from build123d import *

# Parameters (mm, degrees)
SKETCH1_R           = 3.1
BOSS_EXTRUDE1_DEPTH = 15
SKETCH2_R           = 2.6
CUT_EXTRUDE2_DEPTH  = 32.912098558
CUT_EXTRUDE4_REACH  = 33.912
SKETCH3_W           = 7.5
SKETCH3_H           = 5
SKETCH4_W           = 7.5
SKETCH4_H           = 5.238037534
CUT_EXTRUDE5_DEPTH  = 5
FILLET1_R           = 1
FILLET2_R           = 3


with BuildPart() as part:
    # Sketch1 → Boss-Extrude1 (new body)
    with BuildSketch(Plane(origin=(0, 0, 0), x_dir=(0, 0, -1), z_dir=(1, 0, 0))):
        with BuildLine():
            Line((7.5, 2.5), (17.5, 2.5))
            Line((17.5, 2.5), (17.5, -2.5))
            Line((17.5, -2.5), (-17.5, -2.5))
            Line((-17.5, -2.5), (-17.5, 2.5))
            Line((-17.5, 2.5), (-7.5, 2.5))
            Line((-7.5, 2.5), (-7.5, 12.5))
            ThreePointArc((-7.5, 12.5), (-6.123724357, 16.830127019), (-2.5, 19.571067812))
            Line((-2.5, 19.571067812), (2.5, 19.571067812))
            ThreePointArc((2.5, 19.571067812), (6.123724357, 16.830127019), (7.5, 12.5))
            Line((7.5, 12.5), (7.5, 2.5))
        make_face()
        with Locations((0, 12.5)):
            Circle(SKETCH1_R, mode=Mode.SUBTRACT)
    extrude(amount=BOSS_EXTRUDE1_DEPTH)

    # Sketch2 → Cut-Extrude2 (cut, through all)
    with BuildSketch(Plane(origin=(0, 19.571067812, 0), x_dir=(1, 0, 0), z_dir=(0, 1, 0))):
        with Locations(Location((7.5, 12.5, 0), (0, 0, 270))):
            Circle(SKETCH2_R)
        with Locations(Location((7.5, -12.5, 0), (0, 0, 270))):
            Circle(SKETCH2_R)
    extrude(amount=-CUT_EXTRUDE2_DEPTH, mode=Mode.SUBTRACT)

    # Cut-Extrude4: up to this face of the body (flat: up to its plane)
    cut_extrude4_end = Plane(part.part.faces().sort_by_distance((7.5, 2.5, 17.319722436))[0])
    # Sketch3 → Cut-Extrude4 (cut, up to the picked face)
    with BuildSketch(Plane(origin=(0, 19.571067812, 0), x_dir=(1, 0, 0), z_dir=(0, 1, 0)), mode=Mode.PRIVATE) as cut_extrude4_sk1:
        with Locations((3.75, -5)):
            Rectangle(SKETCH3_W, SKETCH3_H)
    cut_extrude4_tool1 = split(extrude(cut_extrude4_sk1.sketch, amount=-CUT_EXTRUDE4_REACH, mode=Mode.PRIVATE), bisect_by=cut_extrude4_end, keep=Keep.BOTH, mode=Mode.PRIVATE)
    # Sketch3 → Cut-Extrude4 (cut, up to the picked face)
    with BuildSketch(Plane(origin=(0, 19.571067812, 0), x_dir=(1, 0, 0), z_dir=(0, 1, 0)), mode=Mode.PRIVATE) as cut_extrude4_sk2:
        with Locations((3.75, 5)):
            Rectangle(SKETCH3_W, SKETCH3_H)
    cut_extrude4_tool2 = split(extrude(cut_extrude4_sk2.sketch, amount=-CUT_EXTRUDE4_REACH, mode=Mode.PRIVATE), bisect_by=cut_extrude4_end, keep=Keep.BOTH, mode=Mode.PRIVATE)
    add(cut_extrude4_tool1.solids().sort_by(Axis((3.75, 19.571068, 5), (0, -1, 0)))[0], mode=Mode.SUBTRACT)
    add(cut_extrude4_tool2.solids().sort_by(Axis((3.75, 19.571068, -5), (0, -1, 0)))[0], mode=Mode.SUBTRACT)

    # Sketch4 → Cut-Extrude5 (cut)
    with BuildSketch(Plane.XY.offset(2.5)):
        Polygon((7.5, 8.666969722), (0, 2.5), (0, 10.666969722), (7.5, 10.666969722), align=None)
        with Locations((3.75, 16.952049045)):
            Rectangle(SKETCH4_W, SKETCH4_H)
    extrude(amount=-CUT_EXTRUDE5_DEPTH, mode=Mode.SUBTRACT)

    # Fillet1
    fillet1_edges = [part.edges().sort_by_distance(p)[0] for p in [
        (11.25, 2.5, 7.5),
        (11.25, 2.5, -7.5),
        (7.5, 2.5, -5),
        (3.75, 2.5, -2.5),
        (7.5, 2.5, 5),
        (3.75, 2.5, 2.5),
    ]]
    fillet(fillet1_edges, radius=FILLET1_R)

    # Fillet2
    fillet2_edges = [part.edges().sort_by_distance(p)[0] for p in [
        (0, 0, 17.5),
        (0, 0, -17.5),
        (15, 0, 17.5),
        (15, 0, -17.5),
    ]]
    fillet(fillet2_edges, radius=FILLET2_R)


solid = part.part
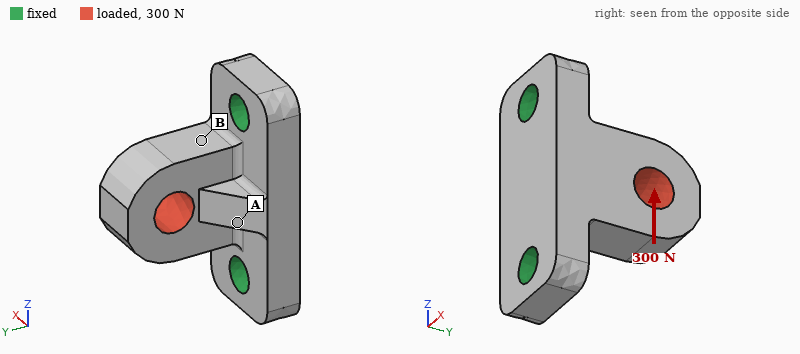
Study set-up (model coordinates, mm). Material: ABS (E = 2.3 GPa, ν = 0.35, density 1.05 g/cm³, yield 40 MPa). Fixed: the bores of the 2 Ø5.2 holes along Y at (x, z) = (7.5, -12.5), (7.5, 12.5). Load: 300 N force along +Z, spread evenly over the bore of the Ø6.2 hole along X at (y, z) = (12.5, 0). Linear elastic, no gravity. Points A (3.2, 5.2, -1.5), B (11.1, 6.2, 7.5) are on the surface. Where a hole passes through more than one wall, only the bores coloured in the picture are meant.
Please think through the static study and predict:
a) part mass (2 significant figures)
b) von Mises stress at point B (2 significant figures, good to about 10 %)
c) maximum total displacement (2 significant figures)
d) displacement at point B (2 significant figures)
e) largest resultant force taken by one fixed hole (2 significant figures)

4.3 g
9.1 MPa
0.19 mm
0.068 mm
250 N
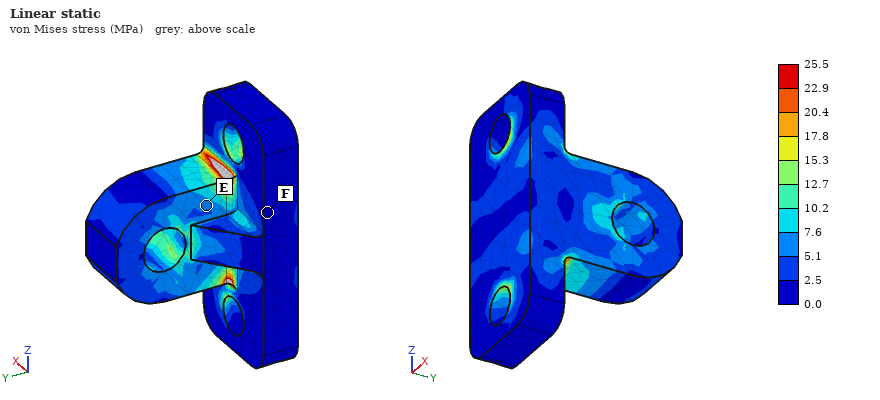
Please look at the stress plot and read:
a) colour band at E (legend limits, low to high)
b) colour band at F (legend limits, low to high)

5.1 to 7.6 MPa
0.0 to 2.5 MPa
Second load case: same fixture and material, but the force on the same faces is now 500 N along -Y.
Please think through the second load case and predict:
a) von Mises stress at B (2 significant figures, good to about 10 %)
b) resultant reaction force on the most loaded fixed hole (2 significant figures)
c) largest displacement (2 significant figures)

7.2 MPa
260 N
0.24 mm
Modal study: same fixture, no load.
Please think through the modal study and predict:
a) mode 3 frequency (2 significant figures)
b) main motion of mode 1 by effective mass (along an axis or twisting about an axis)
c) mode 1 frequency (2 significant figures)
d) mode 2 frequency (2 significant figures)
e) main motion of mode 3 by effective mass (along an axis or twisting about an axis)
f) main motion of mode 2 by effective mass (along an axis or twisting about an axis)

8700 Hz
along X
3400 Hz
6500 Hz
along Y
along Z
